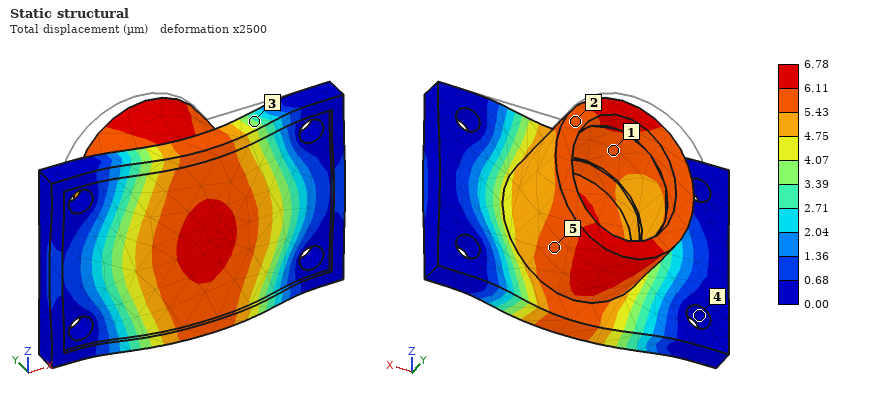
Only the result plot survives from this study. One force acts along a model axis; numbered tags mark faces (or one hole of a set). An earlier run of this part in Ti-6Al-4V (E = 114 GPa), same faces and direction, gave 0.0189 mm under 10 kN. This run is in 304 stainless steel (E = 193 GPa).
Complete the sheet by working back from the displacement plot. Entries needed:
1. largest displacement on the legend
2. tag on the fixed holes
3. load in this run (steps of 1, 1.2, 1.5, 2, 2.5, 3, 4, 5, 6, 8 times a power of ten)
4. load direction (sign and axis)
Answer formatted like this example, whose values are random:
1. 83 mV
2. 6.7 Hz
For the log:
1. 6.78 µm
2. 4
3. 6 kN
4. -Y
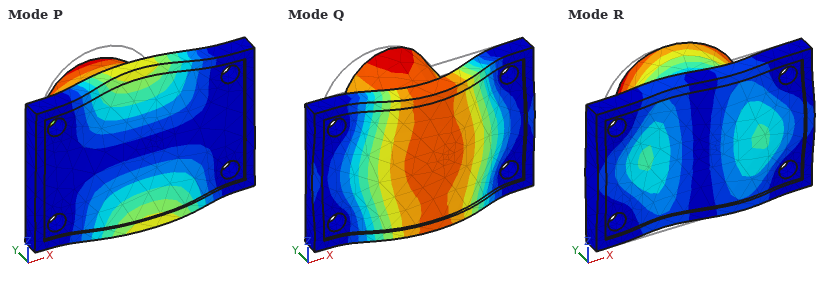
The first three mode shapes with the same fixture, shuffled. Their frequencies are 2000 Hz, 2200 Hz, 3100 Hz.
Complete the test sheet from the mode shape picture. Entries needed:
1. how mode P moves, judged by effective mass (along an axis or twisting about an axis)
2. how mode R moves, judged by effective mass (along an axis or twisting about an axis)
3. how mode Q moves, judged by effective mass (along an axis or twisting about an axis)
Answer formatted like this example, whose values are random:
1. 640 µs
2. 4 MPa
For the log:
1. along Z
2. along X
3. along Y
